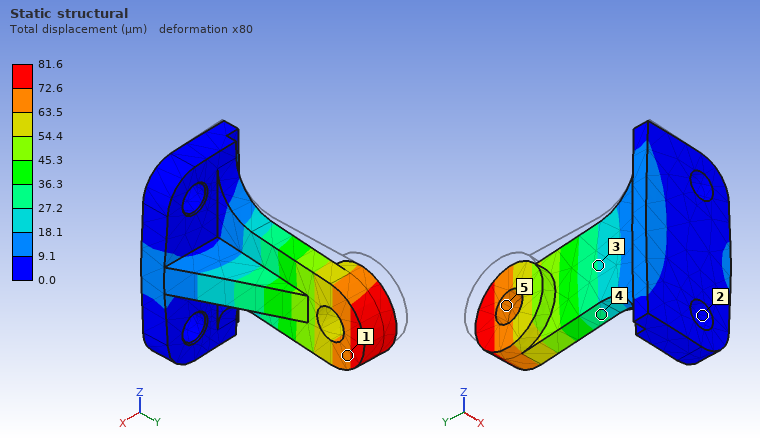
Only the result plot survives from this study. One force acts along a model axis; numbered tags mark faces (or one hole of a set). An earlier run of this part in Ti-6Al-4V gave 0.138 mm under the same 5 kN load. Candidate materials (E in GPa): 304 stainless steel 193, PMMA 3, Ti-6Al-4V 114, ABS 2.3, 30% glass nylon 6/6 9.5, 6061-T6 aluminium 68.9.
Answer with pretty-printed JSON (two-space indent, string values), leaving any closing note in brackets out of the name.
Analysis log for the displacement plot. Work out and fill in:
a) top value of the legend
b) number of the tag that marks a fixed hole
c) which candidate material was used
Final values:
{
  "top value of the legend": "81.6 µm",
  "number of the tag that marks a fixed hole": "2",
  "which candidate material was used": "304 stainless steel"
}
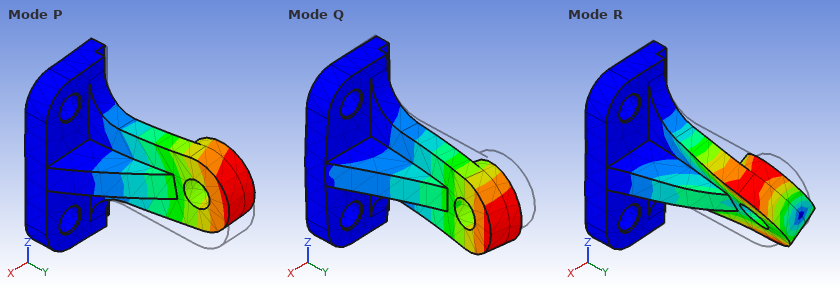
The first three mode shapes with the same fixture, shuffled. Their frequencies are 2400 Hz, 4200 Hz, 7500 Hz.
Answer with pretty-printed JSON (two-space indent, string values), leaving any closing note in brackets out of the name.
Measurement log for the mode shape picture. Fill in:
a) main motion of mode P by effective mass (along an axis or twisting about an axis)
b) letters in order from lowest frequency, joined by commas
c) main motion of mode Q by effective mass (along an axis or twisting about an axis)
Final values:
{
  "main motion of mode P by effective mass": "along Z",
  "letters in order from lowest frequency, joined by commas": "Q, P, R",
  "main motion of mode Q by effective mass": "along X"
}
